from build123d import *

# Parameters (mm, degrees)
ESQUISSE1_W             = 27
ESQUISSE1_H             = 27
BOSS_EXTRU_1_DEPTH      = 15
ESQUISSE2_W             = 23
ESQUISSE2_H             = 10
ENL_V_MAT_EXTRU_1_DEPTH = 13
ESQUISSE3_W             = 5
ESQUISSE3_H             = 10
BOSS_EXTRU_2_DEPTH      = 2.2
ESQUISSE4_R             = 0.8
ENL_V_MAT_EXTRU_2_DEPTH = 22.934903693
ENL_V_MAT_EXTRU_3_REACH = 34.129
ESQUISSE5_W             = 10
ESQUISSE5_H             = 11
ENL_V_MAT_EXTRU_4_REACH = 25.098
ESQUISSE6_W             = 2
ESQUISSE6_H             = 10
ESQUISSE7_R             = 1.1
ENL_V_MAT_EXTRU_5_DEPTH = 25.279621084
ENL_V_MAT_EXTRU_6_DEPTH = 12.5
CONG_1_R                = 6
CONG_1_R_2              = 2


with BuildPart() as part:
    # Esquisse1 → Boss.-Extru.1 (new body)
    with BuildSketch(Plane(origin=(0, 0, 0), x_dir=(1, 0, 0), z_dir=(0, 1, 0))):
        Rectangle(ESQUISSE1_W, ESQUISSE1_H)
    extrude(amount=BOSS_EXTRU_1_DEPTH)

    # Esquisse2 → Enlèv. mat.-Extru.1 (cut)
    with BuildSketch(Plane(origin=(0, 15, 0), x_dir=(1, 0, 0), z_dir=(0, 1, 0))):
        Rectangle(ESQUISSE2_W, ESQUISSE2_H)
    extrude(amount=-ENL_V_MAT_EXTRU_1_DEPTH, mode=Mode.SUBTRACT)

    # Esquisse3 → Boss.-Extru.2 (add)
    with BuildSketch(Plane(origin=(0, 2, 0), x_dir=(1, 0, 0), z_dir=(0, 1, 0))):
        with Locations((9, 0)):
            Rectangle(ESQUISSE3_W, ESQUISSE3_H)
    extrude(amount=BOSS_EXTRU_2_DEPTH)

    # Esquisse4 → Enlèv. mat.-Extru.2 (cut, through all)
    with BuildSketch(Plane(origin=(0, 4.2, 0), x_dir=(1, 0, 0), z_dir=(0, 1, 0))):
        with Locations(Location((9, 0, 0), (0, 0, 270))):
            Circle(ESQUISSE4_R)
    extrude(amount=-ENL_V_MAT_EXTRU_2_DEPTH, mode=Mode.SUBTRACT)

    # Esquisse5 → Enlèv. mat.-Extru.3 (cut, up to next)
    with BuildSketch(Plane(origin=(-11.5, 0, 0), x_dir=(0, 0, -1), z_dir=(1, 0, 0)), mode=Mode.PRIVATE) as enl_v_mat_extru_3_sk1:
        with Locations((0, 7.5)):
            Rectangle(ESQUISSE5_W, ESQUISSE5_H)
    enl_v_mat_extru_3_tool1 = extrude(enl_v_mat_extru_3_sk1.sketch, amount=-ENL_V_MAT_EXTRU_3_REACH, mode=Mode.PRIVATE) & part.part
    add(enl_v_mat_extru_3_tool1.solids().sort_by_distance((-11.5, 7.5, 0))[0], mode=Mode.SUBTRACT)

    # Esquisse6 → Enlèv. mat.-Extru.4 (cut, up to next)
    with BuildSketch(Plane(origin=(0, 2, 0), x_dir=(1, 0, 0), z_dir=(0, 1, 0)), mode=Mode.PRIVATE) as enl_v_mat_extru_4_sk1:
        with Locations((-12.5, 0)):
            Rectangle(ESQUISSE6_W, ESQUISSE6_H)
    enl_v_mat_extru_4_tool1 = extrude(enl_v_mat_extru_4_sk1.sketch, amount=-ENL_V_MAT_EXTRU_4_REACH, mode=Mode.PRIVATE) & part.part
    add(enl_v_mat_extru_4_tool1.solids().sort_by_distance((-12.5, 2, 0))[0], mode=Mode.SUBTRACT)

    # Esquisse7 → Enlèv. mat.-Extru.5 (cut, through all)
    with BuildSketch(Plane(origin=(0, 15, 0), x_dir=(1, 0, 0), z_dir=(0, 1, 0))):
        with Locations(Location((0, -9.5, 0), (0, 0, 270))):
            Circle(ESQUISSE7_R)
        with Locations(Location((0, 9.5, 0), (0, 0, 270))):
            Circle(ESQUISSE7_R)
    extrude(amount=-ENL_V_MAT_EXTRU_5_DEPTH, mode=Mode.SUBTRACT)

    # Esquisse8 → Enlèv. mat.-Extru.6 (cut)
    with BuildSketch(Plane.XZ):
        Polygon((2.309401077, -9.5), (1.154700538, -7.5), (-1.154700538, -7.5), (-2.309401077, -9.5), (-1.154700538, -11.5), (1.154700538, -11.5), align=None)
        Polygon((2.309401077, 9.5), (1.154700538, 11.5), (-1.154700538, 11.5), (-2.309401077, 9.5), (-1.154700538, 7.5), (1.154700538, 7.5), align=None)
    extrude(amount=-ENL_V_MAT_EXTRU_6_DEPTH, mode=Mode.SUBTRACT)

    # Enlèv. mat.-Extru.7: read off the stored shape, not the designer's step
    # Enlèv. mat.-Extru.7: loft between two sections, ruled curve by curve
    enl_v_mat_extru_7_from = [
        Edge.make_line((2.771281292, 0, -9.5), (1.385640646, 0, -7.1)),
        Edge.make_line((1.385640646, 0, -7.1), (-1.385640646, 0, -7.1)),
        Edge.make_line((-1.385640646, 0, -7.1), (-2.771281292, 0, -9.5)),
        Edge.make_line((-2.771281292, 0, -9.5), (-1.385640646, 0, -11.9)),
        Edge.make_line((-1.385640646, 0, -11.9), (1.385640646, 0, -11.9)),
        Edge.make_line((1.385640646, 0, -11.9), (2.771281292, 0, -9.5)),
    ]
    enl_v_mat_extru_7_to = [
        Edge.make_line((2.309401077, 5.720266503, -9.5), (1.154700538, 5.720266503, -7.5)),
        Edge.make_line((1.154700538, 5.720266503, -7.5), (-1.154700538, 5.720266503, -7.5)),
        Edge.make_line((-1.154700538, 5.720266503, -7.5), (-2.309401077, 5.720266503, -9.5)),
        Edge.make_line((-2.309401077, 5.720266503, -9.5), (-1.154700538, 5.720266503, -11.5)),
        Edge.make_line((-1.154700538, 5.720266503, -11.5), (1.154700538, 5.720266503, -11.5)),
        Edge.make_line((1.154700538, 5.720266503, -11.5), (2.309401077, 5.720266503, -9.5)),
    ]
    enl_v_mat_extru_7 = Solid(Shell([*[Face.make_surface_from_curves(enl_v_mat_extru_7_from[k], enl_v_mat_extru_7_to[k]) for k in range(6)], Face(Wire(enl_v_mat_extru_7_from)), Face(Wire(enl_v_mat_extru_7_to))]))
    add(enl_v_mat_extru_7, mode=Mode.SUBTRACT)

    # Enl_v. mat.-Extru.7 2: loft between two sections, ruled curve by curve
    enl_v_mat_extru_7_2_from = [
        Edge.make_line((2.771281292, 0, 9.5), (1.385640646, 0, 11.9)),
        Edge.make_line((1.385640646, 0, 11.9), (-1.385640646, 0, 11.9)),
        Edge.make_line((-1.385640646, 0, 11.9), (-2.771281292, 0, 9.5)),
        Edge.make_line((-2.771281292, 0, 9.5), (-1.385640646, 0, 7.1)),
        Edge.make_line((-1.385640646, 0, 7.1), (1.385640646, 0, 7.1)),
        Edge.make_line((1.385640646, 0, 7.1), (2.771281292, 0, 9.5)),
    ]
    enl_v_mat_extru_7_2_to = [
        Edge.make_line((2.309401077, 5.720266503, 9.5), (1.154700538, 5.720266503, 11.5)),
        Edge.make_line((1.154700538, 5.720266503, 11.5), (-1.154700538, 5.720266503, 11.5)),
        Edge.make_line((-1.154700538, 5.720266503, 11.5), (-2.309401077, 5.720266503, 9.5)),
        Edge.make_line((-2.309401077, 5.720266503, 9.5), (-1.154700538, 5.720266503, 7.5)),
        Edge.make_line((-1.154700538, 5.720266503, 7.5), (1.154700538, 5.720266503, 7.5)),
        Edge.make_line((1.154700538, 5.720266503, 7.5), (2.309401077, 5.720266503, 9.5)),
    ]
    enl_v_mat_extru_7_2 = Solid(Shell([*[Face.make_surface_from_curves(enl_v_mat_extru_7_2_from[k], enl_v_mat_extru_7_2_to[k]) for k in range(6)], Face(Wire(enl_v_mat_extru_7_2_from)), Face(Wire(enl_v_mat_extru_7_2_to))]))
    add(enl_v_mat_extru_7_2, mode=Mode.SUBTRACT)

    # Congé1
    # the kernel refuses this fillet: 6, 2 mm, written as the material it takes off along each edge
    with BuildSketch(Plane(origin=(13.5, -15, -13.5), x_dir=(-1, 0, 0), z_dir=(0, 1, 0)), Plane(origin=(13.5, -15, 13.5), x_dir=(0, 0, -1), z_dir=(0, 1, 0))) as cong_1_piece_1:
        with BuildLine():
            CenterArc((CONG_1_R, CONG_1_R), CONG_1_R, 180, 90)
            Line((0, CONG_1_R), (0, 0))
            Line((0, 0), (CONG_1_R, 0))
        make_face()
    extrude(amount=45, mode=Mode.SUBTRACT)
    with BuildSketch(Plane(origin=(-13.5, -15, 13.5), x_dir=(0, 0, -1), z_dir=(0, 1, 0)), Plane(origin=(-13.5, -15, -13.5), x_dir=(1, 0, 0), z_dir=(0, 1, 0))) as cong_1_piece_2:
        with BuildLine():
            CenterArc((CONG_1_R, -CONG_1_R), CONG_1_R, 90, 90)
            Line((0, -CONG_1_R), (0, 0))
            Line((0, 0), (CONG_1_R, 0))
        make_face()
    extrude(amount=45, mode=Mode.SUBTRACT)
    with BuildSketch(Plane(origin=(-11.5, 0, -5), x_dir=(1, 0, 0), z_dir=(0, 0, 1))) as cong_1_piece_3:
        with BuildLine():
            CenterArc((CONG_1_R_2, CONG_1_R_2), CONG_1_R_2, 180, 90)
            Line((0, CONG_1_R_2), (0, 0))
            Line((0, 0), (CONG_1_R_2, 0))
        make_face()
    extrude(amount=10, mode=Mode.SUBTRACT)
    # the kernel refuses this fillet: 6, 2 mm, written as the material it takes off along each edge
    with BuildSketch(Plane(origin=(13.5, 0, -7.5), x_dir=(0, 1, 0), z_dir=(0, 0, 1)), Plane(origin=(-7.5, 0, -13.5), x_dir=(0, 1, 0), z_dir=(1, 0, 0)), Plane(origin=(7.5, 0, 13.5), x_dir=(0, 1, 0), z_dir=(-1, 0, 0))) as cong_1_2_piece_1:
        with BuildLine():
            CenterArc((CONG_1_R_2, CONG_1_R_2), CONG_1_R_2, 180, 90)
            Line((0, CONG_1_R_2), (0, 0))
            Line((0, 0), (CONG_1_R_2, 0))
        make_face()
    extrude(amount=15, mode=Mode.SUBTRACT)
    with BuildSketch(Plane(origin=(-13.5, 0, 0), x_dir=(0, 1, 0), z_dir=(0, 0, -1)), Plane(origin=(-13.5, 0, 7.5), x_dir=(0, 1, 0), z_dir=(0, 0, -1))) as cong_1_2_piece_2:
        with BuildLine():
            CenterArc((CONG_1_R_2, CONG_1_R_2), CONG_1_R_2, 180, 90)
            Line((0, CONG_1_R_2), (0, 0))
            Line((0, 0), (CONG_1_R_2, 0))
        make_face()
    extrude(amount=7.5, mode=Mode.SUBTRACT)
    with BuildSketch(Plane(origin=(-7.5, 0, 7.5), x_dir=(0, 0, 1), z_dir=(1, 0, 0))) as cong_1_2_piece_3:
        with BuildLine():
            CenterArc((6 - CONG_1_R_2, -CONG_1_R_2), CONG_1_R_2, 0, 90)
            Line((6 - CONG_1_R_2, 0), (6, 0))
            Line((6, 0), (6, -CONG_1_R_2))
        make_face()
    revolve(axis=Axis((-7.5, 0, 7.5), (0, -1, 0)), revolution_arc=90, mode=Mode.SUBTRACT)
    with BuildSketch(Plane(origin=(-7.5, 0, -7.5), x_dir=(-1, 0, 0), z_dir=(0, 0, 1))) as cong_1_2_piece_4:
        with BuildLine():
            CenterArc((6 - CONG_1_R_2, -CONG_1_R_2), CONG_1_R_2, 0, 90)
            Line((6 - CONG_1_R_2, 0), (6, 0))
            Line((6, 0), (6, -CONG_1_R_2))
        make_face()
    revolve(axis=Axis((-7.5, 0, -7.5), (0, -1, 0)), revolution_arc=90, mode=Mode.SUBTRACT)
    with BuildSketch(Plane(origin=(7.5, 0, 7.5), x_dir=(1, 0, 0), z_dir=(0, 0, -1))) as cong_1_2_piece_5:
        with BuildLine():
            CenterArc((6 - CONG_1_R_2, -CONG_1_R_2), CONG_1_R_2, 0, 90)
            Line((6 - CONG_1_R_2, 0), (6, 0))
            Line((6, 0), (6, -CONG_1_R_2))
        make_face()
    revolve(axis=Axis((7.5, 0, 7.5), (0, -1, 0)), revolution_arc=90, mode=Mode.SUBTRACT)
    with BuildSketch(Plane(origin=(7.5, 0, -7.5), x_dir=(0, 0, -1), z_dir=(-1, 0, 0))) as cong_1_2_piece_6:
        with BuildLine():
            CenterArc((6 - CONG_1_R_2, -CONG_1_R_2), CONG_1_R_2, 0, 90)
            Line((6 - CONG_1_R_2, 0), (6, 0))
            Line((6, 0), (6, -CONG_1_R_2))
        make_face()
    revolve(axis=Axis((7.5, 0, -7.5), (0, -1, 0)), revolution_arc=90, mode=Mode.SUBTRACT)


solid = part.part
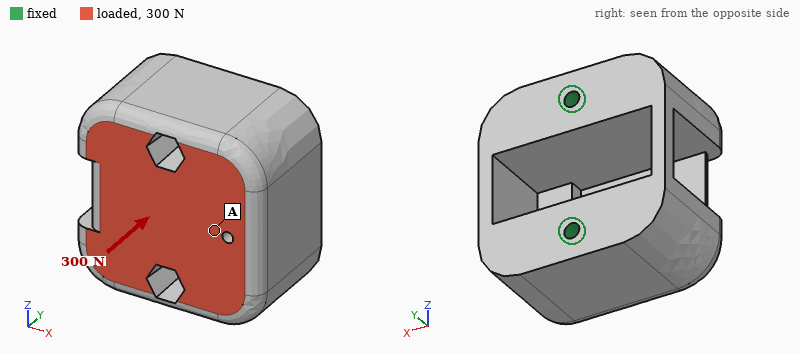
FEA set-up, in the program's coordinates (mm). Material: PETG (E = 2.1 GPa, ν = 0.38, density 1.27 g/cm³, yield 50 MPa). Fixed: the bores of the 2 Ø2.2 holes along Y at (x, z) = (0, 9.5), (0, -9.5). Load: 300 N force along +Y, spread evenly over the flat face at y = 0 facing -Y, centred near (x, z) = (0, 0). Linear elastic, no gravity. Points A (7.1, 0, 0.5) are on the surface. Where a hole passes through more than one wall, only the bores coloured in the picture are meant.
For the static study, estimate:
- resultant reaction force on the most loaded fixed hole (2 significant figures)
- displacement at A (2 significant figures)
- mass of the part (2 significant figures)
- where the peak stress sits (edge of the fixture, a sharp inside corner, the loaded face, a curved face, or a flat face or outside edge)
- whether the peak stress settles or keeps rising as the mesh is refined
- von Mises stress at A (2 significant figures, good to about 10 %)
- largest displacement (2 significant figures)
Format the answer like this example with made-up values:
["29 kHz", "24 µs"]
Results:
["150 N", "67 µm", "8.7 g", "edge of the fixture", "keeps rising", "3.1 MPa", "72 µm"]
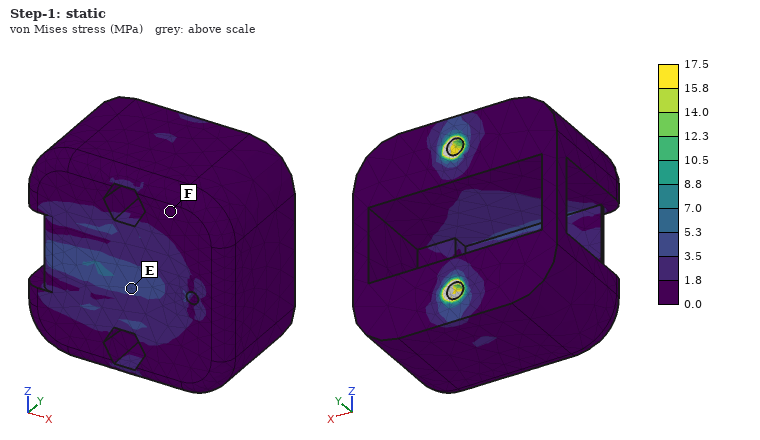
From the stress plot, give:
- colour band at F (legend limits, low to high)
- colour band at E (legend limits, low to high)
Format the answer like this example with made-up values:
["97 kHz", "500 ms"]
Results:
["0.0 to 1.8 MPa", "3.5 to 5.3 MPa"]
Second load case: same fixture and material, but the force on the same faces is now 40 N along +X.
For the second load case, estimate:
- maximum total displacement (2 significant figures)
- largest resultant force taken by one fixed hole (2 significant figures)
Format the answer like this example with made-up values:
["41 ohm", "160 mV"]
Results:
["0.20 mm", "20 N"]
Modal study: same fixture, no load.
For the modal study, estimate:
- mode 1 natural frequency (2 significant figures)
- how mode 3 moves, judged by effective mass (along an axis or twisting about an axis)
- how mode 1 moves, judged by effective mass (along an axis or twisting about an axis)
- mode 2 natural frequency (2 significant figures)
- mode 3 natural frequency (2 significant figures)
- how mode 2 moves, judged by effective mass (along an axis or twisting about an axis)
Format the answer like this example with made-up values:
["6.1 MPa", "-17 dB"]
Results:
["1100 Hz", "along Z", "along X", "2200 Hz", "3200 Hz", "along Z"]
